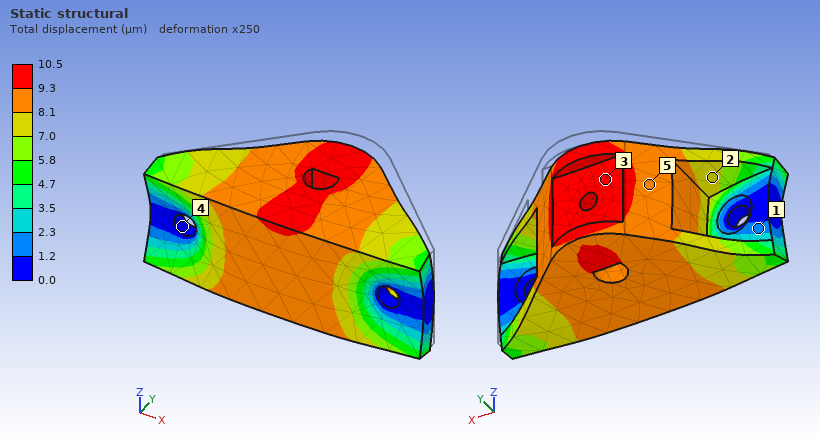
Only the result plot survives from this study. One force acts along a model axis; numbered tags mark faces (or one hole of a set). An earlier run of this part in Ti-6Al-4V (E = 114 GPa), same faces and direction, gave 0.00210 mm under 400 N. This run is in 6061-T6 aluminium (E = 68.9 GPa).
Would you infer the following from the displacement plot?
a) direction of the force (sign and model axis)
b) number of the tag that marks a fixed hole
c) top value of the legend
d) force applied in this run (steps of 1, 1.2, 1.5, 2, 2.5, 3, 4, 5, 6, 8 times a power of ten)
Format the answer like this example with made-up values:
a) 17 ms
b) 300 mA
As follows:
a) -Y
b) 4
c) 10.5 µm
d) 1.2 kN
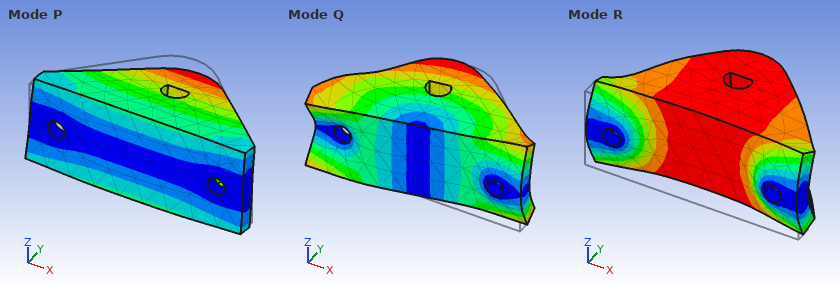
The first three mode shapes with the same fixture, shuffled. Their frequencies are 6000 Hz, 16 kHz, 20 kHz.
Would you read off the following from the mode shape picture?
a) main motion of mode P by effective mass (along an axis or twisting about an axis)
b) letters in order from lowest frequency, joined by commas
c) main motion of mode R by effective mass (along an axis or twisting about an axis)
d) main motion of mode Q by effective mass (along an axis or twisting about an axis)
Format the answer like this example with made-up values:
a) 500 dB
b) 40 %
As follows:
a) along Z
b) P, R, Q
c) along Y
d) along X
